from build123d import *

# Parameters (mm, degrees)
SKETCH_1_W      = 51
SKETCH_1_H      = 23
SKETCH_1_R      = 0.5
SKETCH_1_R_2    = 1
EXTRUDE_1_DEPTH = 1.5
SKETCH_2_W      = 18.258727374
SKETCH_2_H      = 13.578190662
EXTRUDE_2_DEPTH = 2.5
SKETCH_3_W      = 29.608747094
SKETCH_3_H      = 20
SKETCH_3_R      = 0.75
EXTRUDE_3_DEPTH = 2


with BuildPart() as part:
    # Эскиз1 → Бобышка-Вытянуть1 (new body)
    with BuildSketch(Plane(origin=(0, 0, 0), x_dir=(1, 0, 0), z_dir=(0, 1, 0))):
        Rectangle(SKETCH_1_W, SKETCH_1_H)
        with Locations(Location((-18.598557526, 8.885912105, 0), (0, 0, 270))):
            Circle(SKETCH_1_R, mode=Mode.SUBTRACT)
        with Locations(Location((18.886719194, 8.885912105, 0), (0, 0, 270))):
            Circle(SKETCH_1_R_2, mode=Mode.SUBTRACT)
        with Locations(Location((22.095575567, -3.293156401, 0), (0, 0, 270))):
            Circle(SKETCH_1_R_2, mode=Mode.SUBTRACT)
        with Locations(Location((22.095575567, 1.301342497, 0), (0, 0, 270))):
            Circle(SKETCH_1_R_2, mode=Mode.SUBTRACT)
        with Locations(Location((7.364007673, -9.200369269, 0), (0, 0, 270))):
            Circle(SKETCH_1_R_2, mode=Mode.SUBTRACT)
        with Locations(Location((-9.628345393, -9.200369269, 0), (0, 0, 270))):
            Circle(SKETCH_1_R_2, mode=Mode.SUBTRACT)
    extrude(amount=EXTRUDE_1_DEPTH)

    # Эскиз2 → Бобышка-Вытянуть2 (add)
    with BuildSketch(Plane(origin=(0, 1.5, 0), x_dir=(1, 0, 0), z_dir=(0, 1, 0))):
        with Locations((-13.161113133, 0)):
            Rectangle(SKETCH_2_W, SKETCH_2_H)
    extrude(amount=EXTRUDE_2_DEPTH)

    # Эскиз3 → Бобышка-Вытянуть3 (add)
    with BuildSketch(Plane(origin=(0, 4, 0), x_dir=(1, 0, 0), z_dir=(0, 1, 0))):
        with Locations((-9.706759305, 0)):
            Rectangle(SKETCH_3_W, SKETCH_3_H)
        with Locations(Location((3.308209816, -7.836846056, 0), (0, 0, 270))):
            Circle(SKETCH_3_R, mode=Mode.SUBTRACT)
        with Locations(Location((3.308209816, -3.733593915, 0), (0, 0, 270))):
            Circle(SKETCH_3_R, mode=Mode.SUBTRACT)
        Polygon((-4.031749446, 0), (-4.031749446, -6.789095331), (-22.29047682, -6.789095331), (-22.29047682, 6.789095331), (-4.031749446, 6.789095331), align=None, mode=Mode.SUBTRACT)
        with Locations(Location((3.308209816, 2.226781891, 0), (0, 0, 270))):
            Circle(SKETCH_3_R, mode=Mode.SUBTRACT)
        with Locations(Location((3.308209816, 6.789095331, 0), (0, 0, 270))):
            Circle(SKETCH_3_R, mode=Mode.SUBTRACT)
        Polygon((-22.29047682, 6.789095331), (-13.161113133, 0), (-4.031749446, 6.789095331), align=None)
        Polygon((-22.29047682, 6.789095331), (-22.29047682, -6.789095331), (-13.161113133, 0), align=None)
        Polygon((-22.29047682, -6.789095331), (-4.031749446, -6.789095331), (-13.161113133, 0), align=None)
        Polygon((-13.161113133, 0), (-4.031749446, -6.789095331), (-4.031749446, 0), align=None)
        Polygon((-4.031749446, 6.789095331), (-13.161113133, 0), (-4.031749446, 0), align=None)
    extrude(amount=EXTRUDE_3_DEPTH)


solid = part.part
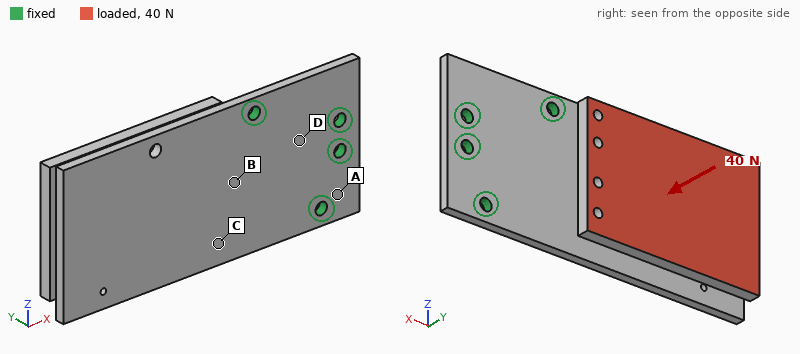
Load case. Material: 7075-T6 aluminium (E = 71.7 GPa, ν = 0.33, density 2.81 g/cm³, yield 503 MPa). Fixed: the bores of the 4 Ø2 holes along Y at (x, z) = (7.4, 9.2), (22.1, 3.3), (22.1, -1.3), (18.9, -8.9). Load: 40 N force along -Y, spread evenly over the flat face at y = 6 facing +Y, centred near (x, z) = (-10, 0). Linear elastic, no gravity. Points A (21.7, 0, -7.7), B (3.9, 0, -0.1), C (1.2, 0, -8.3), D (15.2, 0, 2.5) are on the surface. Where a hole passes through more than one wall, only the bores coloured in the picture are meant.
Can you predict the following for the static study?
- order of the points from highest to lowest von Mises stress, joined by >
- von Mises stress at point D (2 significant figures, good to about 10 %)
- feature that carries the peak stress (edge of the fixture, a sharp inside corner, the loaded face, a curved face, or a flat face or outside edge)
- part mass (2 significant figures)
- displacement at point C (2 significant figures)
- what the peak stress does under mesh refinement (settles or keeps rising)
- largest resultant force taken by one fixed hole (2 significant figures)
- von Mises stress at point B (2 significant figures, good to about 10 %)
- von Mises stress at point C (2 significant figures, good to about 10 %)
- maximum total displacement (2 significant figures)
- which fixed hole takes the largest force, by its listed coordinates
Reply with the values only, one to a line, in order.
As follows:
B > C > D > A
20 MPa
edge of the fixture
9.9 g
0.12 mm
keeps rising
53 N
52 MPa
39 MPa
0.55 mm
(7.4, 9.2)
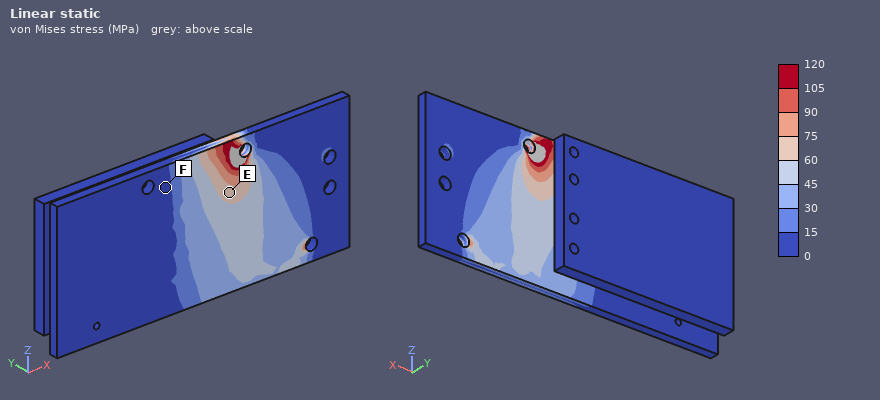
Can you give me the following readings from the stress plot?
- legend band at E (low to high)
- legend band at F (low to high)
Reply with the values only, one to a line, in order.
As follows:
60 to 75 MPa
0 to 15 MPa
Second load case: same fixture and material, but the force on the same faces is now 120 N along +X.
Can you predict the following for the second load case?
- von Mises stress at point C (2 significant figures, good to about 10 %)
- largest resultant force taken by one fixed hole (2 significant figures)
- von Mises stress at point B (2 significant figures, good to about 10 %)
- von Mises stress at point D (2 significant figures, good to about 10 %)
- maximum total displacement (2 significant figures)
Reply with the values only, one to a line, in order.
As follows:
57 MPa
48 N
56 MPa
10 MPa
0.59 mm
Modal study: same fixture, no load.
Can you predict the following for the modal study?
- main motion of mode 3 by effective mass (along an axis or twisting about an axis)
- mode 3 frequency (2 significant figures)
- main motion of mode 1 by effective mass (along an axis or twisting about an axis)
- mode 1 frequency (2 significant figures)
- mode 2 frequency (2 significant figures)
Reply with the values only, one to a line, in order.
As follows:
along Y
4700 Hz
along Y
600 Hz
2300 Hz
